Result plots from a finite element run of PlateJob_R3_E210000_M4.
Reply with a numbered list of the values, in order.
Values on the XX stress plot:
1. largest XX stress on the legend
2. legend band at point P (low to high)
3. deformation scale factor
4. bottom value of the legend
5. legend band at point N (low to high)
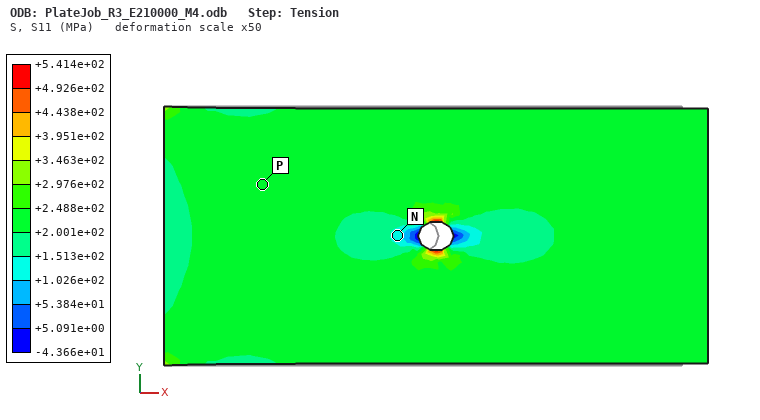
1. +5.414e+02 MPa
2. +2.001e+02 to +2.488e+02 MPa
3. 50
4. -4.366e+01 MPa
5. +1.026e+02 to +1.513e+02 MPa
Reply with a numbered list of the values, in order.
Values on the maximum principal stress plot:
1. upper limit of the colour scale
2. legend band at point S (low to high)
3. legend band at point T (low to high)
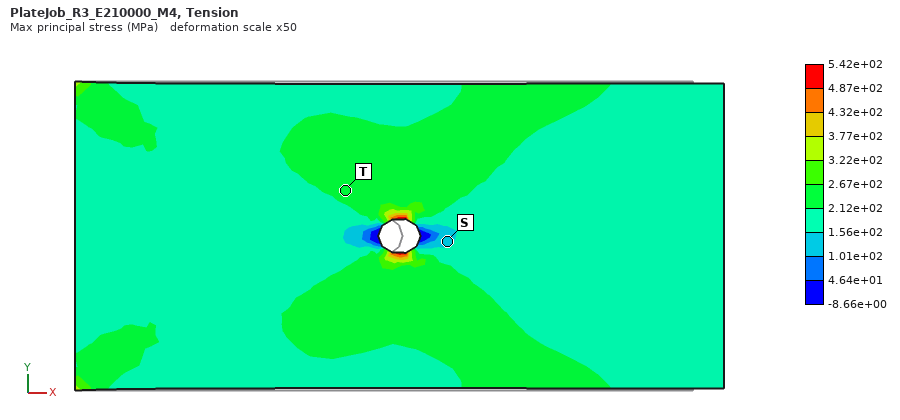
1. 5.42e+02 MPa
2. 1.01e+02 to 1.56e+02 MPa
3. 2.12e+02 to 2.67e+02 MPa
